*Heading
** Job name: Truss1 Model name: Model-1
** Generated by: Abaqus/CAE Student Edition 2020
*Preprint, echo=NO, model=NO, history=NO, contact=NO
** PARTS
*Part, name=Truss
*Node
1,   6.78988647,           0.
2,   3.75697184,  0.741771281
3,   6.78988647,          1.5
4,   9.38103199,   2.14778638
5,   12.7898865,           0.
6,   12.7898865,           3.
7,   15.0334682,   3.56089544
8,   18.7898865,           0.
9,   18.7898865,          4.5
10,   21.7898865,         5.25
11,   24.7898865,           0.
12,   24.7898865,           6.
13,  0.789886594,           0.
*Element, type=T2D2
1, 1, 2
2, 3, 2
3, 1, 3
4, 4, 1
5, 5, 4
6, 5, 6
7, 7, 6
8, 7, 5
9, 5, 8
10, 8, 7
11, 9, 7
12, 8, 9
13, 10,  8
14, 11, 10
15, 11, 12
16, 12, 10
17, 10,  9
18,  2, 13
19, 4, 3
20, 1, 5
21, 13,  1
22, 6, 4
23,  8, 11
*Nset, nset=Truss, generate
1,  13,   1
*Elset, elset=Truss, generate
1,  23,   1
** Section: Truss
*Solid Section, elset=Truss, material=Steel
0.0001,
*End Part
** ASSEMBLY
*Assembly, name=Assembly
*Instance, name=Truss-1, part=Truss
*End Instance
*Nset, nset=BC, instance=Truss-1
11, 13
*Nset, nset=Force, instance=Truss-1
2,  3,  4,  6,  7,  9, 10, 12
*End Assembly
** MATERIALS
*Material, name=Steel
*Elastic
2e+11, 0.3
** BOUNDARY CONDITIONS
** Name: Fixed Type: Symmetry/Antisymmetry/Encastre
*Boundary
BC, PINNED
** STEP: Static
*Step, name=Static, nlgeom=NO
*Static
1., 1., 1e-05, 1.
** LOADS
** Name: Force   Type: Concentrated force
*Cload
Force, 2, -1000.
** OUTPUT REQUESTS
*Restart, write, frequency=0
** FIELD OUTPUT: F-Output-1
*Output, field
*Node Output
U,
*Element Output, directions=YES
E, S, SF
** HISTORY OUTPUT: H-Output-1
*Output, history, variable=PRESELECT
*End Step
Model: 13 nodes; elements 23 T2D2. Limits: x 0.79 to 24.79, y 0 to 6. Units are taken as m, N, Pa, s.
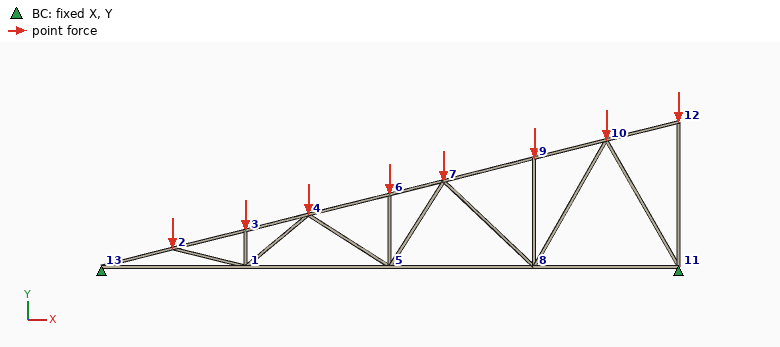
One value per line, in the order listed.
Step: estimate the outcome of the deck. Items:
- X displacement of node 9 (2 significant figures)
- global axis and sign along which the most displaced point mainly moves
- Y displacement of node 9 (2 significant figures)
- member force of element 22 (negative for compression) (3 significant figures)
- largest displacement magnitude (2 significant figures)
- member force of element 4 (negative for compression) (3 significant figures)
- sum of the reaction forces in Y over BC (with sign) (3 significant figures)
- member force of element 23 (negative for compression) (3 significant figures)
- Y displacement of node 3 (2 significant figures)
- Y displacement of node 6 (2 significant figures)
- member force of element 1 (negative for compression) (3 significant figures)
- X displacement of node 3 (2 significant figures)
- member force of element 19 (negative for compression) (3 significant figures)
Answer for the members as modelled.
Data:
-0.0059 m
-Y
-0.014 m
-8300 N
0.030 m
2340 N
8000 N
-6290 N
-0.030 m
-0.025 m
-2080 N
0.0031 m
-12600 N
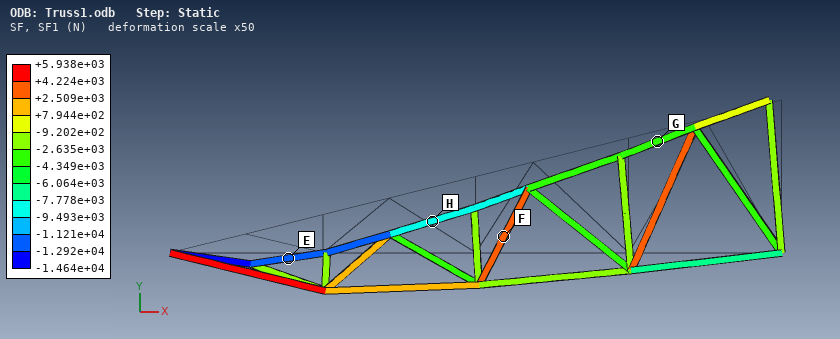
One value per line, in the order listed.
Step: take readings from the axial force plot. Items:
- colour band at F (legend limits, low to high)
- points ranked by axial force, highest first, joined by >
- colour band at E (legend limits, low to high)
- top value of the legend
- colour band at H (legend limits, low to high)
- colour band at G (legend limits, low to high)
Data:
+2.509e+03 to +4.224e+03 N
F > G > H > E
-1.292e+04 to -1.121e+04 N
+5.938e+03 N
-9.493e+03 to -7.778e+03 N
-4.349e+03 to -2.635e+03 N
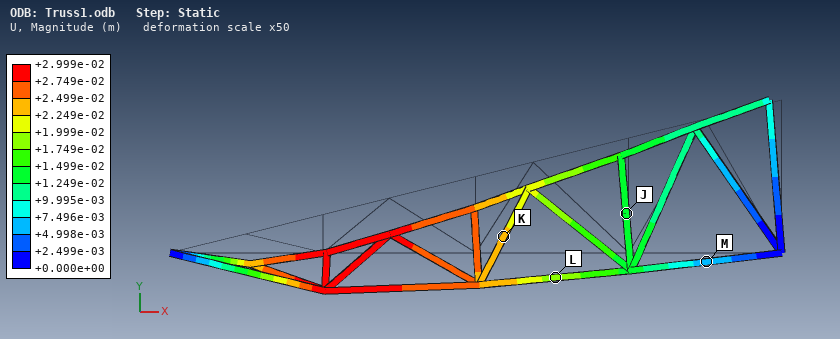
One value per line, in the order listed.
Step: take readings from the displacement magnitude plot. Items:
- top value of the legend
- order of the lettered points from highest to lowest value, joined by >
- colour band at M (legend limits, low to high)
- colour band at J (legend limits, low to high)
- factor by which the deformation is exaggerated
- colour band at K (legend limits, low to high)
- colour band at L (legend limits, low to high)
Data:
+2.999e-02 m
K > L > J > M
+4.998e-03 to +7.496e-03 m
+1.249e-02 to +1.499e-02 m
50
+2.249e-02 to +2.499e-02 m
+1.749e-02 to +1.999e-02 m
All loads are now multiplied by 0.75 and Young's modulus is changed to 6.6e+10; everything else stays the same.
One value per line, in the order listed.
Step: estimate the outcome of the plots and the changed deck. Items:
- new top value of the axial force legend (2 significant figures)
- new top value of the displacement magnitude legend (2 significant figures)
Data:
4500 N
0.068 m
